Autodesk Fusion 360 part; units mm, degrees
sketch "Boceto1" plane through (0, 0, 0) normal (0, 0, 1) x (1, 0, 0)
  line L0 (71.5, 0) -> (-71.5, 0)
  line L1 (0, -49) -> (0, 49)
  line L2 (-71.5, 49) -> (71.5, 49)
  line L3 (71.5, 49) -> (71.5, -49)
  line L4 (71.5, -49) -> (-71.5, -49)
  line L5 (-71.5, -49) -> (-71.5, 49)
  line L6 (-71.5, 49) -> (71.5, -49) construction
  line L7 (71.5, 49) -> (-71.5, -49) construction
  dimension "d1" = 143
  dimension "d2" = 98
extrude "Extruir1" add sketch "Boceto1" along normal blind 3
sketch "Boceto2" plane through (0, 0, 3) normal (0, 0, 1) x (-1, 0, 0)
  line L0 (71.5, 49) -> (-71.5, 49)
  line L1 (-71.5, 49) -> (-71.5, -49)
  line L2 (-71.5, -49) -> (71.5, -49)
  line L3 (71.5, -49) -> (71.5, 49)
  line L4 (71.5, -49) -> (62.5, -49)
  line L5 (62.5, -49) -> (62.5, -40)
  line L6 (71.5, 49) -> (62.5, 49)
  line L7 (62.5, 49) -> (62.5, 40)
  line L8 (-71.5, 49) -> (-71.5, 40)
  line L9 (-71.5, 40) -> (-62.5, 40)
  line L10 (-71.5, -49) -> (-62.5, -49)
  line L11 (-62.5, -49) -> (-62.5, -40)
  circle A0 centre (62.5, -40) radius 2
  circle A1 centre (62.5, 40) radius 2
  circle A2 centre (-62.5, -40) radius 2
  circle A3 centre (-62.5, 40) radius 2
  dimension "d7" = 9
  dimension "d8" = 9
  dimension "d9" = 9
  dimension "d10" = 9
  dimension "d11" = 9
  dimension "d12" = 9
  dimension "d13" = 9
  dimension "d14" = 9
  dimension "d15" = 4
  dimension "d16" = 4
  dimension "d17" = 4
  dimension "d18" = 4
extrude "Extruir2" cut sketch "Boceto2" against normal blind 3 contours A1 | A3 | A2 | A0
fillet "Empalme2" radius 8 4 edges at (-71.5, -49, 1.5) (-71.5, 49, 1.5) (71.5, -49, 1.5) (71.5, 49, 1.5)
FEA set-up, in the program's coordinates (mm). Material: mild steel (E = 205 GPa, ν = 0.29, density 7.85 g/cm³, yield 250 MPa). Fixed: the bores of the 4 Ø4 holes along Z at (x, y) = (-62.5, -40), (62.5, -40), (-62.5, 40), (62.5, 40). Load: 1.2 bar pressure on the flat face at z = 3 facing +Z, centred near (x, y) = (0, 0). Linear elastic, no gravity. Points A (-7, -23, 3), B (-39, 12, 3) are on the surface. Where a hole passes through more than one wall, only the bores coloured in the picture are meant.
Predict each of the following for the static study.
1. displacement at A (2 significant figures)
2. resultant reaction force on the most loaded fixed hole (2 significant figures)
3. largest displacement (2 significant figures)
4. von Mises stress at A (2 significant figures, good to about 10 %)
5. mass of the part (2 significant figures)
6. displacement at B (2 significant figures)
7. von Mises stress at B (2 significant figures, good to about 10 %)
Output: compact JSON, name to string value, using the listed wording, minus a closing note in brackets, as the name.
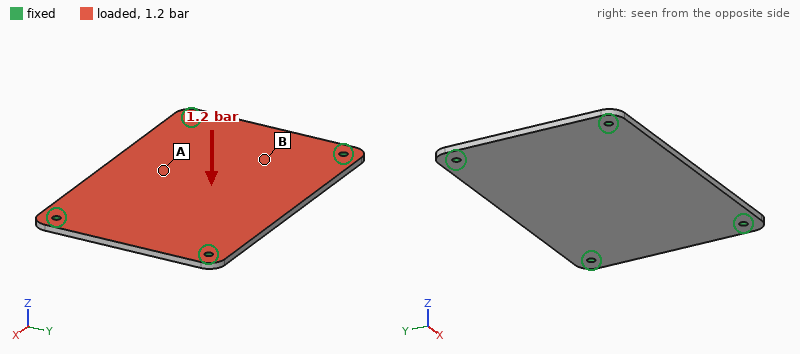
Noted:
{"displacement at A": "0.24 mm", "resultant reaction force on the most loaded fixed hole": "420 N", "largest displacement": "0.26 mm", "von Mises stress at A": "55 MPa", "mass of the part": "330 g", "displacement at B": "0.14 mm", "von Mises stress at B": "26 MPa"}
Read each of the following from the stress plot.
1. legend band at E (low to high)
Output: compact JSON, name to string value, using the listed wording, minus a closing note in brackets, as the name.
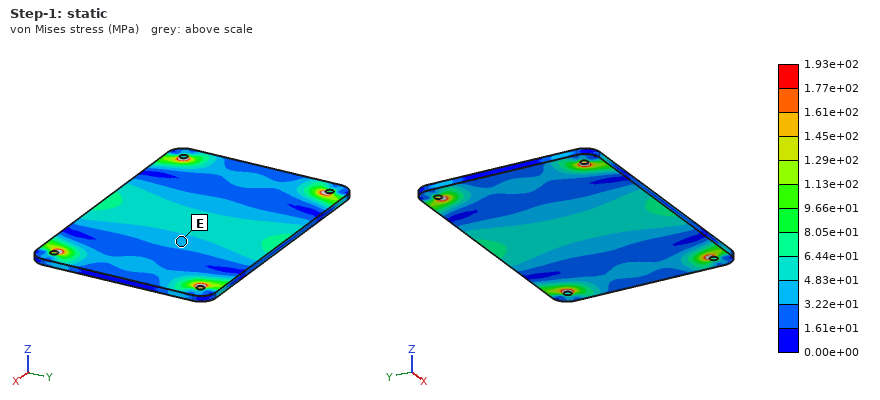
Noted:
{"legend band at E": "3.22e+01 to 4.83e+01 MPa"}
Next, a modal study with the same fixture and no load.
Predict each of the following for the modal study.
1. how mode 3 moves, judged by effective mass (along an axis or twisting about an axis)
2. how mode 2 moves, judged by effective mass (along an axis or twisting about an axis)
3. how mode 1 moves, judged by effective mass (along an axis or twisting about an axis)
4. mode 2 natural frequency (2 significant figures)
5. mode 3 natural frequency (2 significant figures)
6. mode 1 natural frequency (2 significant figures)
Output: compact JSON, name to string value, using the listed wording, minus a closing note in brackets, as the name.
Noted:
{"how mode 3 moves, judged by effective mass": "twisting about Y", "how mode 2 moves, judged by effective mass": "twisting about X", "how mode 1 moves, judged by effective mass": "along Z", "mode 2 natural frequency": "1300 Hz", "mode 3 natural frequency": "2100 Hz", "mode 1 natural frequency": "820 Hz"}
